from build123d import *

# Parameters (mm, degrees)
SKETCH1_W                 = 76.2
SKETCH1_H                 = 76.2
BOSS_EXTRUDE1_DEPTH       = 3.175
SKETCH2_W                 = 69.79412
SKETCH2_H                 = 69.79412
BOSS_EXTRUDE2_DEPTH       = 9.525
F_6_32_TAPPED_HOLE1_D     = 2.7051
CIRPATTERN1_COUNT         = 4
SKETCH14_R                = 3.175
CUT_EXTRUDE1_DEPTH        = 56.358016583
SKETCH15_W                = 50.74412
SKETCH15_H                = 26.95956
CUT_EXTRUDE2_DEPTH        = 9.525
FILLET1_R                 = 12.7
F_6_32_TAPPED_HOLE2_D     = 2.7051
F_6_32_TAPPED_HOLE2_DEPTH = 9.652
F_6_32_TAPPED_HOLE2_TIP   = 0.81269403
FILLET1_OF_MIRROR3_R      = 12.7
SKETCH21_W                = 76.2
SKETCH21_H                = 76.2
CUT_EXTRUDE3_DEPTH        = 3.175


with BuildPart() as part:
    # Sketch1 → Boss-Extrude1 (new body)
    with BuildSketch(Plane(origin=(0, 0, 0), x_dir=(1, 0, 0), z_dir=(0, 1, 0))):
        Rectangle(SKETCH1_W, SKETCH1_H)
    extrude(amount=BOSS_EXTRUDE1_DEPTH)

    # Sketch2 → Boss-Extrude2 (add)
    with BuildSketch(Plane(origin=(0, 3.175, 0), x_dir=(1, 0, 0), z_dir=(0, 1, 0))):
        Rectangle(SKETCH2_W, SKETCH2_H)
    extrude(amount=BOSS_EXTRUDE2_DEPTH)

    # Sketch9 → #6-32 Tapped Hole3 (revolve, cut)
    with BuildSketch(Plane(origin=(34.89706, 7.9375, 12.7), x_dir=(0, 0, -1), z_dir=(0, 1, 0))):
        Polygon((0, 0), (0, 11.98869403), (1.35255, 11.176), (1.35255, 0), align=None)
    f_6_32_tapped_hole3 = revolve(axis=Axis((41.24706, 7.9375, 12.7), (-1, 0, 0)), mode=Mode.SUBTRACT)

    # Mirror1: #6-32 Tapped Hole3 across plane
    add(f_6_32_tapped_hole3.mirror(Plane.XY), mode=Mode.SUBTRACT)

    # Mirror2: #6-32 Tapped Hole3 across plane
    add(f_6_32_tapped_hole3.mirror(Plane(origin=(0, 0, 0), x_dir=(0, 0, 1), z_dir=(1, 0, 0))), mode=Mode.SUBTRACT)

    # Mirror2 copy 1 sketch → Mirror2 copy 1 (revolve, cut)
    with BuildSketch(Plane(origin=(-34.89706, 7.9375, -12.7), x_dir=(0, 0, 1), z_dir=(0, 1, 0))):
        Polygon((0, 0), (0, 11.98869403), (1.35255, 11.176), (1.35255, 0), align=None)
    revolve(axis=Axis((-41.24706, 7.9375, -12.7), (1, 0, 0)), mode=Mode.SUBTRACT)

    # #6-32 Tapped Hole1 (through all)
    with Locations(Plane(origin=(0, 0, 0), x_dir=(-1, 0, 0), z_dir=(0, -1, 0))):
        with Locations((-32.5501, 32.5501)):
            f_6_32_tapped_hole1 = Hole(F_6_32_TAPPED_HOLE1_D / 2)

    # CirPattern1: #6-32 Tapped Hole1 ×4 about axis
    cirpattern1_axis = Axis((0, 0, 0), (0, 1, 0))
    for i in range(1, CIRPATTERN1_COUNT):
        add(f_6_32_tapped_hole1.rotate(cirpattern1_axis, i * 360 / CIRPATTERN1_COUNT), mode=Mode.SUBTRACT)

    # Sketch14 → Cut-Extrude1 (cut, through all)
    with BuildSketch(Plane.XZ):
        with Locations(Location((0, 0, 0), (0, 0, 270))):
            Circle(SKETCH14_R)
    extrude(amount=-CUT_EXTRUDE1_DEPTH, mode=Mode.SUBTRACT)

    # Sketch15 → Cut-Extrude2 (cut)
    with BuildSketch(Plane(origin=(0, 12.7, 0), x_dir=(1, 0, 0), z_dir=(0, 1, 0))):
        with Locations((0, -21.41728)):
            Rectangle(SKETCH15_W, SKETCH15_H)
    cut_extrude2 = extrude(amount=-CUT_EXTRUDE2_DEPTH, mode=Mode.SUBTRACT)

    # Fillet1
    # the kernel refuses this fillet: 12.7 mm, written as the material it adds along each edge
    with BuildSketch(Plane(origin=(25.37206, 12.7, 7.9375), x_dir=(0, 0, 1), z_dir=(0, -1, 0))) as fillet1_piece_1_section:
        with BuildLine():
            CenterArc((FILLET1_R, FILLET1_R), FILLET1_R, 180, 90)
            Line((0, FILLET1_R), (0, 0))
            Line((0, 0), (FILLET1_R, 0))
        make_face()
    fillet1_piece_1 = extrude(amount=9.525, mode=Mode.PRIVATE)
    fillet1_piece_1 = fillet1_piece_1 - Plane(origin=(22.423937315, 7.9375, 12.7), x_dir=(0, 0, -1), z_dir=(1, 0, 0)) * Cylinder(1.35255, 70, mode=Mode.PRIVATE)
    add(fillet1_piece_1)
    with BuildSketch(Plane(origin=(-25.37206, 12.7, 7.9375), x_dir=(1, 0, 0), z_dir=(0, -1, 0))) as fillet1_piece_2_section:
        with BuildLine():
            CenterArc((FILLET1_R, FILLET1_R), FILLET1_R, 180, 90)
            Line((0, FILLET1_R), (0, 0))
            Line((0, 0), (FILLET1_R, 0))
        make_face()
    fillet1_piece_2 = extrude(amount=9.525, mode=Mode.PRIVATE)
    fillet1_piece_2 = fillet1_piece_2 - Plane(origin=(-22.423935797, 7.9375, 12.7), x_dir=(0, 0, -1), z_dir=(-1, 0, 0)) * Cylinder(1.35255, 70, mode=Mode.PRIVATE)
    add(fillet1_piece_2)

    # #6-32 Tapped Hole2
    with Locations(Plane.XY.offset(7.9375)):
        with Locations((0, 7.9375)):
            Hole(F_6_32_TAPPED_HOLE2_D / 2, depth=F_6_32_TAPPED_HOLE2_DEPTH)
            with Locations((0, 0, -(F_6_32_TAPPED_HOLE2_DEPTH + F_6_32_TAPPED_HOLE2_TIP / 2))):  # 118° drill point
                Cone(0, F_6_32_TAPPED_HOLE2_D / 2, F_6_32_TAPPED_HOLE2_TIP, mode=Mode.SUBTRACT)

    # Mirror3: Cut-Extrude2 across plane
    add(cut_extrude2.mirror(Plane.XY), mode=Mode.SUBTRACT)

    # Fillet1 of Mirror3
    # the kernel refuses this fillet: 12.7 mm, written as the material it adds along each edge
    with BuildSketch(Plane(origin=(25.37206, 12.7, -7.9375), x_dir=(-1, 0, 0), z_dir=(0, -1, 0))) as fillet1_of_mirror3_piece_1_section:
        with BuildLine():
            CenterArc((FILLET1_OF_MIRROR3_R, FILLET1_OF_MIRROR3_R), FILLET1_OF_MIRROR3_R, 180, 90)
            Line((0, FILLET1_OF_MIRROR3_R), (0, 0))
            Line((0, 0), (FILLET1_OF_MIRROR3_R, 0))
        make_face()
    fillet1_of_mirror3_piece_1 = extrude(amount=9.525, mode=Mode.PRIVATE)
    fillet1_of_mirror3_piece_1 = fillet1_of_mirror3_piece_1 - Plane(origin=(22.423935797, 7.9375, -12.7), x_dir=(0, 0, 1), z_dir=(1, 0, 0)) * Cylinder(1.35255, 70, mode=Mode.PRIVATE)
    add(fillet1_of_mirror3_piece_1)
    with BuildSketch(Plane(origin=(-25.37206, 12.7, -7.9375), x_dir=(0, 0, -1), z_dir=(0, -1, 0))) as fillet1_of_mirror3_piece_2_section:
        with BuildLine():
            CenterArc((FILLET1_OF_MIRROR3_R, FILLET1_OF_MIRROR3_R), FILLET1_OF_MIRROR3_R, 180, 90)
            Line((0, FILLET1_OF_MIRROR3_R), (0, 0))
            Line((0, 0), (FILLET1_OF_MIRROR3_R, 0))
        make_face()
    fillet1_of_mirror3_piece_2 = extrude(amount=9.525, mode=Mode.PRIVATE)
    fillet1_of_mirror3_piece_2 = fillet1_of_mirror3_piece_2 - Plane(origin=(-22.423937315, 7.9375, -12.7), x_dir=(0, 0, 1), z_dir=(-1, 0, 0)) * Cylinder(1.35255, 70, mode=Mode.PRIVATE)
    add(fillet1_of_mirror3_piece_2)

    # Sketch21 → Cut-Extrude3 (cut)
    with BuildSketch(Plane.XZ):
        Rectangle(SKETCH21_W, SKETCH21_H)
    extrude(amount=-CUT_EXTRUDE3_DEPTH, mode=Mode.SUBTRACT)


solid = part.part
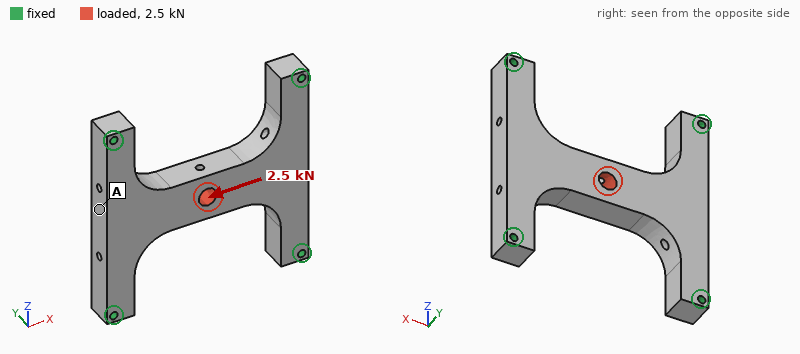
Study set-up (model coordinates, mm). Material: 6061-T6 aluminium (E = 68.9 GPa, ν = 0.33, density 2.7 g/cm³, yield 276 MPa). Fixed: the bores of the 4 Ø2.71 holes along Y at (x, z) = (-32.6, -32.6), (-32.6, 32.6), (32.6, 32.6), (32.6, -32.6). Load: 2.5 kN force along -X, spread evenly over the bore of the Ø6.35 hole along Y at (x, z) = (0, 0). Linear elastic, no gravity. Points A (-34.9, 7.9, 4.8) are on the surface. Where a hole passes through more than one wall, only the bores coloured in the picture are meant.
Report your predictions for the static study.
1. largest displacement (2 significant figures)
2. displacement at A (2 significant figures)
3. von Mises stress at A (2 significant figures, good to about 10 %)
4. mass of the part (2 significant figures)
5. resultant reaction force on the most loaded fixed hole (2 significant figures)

29 µm
27 µm
15 MPa
56 g
1.0 kN
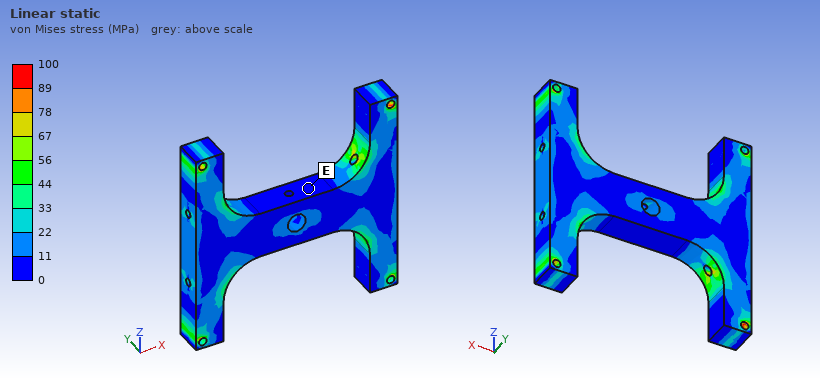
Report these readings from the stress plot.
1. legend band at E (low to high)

0 to 11 MPa
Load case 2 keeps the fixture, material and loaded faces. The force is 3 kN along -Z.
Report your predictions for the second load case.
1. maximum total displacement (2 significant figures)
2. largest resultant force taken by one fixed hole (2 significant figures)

29 µm
890 N
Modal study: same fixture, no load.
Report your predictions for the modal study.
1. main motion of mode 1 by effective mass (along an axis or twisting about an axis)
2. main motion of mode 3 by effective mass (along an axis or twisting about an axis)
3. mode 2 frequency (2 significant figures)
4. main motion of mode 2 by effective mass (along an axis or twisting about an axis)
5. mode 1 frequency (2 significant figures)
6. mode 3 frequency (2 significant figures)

along Y
twisting about Z
7600 Hz
along X
5400 Hz
9000 Hz
